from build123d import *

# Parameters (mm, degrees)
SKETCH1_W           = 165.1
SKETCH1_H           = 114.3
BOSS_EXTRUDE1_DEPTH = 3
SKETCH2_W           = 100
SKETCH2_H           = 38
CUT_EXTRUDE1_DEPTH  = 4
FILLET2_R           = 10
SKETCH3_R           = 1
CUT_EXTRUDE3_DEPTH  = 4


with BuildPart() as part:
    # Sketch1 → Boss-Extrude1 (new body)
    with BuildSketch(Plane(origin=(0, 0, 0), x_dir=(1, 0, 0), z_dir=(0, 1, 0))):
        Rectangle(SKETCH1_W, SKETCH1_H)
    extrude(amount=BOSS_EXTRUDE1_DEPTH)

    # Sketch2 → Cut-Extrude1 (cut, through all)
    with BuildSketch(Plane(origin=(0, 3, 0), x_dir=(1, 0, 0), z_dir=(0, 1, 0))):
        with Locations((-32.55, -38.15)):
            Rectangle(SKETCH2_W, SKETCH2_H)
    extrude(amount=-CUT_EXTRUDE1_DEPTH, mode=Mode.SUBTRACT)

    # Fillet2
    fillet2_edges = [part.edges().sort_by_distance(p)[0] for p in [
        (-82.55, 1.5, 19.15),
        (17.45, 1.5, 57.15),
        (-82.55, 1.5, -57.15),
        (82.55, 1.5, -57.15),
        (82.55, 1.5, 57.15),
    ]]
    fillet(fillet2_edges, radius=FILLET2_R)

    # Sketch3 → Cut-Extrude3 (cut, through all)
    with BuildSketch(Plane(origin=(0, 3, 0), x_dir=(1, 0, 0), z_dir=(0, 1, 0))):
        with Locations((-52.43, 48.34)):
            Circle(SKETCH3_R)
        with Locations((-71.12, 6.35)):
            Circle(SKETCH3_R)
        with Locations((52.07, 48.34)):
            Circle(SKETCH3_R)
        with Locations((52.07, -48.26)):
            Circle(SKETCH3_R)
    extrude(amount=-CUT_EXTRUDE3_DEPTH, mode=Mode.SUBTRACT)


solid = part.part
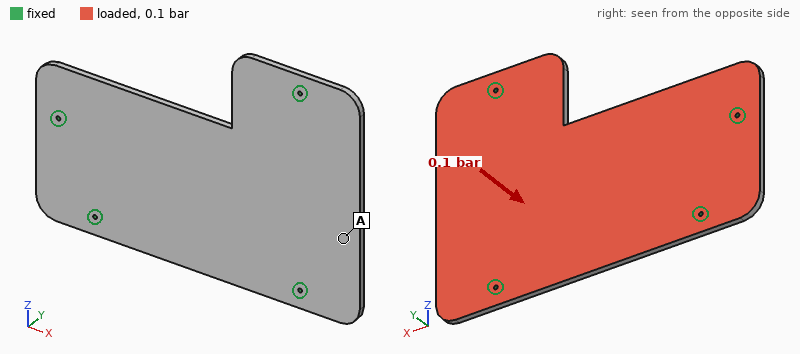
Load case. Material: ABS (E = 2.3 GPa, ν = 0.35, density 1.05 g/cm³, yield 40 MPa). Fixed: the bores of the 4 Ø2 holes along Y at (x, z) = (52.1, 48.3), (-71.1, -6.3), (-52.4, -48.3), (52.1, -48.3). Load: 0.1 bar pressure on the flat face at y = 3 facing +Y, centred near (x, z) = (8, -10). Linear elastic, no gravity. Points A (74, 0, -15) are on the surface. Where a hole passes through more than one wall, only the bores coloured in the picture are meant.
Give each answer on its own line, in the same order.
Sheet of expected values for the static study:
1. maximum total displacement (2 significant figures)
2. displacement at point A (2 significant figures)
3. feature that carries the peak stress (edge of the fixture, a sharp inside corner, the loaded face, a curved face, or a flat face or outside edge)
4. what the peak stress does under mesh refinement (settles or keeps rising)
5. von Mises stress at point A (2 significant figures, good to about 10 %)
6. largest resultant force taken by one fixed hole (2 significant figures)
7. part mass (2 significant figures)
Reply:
2.0 mm
0.70 mm
edge of the fixture
keeps rising
2.8 MPa
46 N
47 g
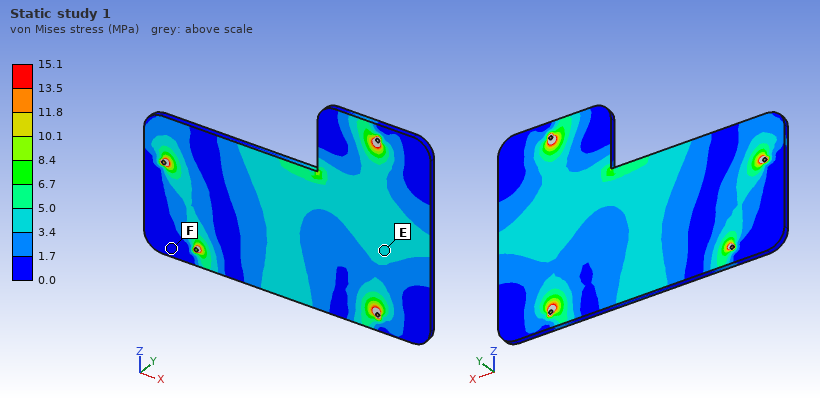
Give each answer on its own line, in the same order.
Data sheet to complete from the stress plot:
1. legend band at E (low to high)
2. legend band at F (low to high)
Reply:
3.4 to 5.0 MPa
0.0 to 1.7 MPa
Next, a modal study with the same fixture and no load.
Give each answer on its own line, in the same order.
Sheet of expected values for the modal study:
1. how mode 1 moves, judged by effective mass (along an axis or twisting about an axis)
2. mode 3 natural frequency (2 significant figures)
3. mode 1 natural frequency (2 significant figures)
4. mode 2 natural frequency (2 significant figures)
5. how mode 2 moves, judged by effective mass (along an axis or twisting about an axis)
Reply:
along Y
470 Hz
250 Hz
350 Hz
along Y
